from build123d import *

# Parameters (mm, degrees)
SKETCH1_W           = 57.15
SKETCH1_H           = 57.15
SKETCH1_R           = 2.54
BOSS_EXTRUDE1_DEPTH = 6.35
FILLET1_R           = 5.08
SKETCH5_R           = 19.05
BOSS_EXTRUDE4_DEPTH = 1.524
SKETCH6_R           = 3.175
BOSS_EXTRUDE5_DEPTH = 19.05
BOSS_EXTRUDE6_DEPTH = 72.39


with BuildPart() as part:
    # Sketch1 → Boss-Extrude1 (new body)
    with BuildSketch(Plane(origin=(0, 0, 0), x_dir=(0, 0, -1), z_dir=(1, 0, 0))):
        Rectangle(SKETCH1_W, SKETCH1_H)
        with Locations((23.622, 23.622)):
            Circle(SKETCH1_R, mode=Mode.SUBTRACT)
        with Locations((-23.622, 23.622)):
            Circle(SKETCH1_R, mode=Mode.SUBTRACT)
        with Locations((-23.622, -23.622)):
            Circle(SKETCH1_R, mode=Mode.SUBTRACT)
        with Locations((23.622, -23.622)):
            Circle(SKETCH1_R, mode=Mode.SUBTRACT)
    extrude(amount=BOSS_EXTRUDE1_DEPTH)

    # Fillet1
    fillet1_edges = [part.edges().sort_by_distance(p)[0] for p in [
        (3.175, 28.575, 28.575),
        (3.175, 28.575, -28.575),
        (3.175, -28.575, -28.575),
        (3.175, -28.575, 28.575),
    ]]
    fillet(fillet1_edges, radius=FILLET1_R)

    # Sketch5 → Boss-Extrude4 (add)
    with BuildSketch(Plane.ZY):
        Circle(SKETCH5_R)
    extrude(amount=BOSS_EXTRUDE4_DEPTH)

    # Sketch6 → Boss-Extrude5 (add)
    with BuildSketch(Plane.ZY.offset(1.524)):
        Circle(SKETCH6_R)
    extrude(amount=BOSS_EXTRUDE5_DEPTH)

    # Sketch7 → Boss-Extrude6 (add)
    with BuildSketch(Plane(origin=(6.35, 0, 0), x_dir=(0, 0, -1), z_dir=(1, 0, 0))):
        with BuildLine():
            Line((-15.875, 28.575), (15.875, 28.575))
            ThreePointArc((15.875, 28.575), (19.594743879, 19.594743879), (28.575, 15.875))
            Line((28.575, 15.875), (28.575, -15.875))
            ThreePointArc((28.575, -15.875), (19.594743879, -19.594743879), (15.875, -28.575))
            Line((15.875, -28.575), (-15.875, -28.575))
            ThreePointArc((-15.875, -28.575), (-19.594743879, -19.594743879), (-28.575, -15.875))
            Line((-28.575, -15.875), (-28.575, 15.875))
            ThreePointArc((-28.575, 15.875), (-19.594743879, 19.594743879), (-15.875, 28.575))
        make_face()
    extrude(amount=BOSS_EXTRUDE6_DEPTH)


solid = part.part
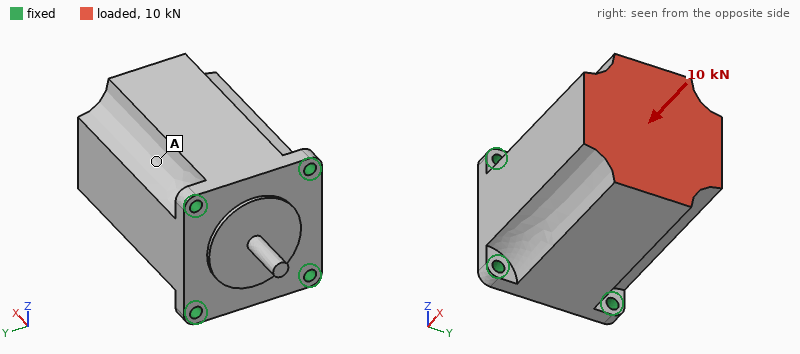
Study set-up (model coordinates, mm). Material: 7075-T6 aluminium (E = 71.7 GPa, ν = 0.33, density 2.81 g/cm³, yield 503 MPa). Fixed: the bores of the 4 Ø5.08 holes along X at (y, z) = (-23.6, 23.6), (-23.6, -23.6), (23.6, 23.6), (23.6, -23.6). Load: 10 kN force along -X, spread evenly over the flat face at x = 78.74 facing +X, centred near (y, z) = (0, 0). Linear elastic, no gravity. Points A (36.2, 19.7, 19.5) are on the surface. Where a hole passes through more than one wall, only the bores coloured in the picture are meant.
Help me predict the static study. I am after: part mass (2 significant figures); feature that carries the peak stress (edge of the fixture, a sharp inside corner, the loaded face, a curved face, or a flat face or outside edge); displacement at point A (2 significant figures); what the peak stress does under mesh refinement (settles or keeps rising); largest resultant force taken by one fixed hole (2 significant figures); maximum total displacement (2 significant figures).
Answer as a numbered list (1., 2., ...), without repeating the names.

1. 620 g
2. edge of the fixture
3. 12 µm
4. keeps rising
5. 2.7 kN
6. 14 µm
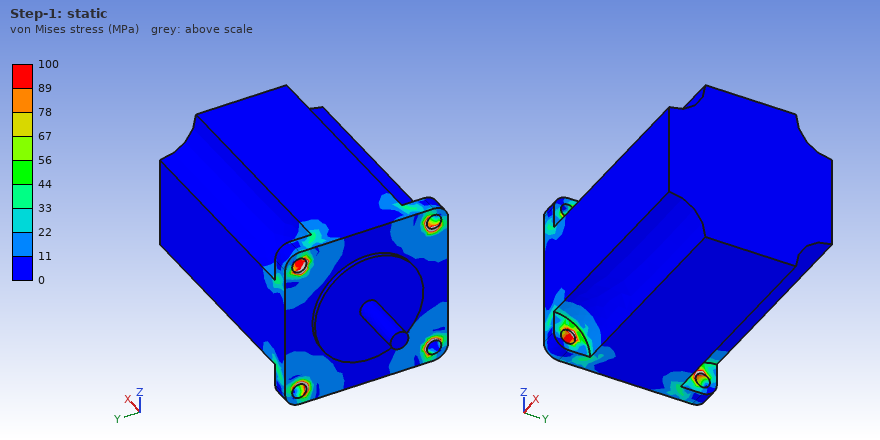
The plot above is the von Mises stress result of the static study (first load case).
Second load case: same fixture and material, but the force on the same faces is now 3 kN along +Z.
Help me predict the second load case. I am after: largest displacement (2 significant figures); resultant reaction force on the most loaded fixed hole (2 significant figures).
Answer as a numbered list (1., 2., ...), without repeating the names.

1. 53 µm
2. 2.8 kN
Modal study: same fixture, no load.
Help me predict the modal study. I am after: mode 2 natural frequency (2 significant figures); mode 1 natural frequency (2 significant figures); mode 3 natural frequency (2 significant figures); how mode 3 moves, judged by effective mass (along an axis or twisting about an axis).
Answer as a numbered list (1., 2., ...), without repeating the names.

1. 2700 Hz
2. 2700 Hz
3. 6000 Hz
4. along X
